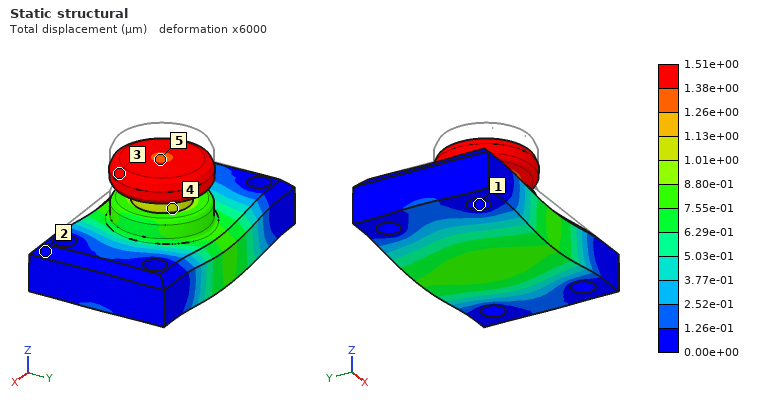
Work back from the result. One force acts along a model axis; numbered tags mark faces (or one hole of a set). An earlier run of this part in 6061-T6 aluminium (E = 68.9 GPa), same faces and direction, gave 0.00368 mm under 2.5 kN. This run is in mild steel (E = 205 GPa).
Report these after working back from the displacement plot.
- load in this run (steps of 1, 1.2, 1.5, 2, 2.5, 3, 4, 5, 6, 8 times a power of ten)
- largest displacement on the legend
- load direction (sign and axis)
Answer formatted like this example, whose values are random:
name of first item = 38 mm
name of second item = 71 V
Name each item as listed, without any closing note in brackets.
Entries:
load in this run = 3 kN
largest displacement on the legend = 1.51e+00 µm
load direction = -Z
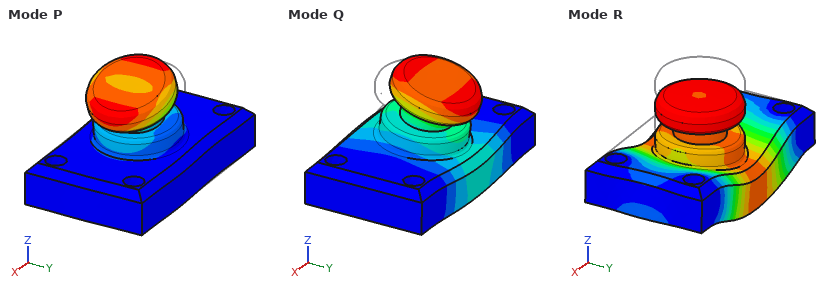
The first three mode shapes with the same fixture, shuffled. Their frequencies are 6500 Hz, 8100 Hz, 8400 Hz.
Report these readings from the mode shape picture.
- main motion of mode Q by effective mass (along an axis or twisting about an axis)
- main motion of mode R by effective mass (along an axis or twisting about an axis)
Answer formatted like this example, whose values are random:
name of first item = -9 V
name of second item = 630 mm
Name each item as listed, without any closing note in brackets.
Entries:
main motion of mode Q by effective mass = along Y
main motion of mode R by effective mass = along Z
